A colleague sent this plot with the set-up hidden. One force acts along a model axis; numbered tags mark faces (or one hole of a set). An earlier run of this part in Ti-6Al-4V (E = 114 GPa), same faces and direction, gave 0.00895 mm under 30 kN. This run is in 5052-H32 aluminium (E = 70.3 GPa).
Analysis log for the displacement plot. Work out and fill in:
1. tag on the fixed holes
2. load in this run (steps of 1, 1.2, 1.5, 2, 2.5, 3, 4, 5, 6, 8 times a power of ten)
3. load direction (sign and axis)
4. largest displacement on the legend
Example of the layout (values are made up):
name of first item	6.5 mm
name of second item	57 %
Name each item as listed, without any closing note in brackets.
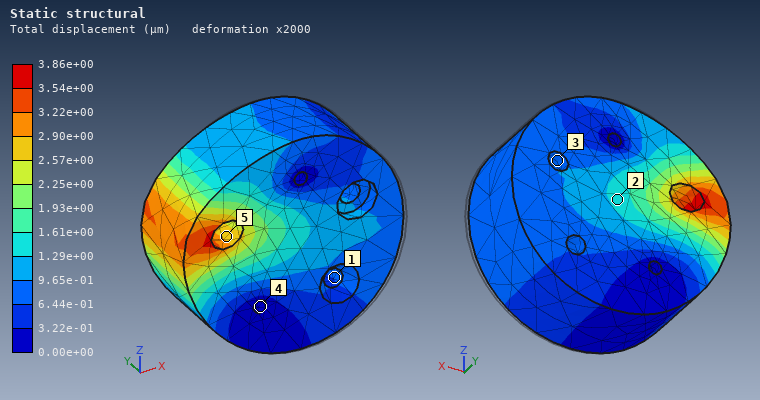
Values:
tag on the fixed holes	4
load in this run	8 kN
load direction	-X
largest displacement on the legend	3.86e+00 µm
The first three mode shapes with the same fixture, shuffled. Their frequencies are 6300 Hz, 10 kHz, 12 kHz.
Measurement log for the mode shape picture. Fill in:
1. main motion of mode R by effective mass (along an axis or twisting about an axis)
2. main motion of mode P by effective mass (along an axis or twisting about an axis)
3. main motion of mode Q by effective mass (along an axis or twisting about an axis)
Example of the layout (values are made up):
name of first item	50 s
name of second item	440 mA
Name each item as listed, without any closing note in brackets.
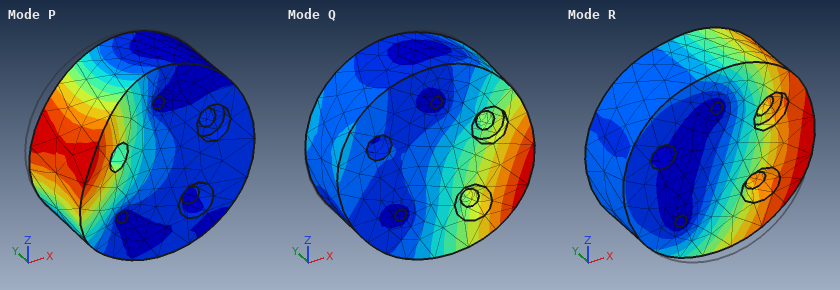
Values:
main motion of mode R by effective mass	along Z
main motion of mode P by effective mass	along Y
main motion of mode Q by effective mass	along Y
